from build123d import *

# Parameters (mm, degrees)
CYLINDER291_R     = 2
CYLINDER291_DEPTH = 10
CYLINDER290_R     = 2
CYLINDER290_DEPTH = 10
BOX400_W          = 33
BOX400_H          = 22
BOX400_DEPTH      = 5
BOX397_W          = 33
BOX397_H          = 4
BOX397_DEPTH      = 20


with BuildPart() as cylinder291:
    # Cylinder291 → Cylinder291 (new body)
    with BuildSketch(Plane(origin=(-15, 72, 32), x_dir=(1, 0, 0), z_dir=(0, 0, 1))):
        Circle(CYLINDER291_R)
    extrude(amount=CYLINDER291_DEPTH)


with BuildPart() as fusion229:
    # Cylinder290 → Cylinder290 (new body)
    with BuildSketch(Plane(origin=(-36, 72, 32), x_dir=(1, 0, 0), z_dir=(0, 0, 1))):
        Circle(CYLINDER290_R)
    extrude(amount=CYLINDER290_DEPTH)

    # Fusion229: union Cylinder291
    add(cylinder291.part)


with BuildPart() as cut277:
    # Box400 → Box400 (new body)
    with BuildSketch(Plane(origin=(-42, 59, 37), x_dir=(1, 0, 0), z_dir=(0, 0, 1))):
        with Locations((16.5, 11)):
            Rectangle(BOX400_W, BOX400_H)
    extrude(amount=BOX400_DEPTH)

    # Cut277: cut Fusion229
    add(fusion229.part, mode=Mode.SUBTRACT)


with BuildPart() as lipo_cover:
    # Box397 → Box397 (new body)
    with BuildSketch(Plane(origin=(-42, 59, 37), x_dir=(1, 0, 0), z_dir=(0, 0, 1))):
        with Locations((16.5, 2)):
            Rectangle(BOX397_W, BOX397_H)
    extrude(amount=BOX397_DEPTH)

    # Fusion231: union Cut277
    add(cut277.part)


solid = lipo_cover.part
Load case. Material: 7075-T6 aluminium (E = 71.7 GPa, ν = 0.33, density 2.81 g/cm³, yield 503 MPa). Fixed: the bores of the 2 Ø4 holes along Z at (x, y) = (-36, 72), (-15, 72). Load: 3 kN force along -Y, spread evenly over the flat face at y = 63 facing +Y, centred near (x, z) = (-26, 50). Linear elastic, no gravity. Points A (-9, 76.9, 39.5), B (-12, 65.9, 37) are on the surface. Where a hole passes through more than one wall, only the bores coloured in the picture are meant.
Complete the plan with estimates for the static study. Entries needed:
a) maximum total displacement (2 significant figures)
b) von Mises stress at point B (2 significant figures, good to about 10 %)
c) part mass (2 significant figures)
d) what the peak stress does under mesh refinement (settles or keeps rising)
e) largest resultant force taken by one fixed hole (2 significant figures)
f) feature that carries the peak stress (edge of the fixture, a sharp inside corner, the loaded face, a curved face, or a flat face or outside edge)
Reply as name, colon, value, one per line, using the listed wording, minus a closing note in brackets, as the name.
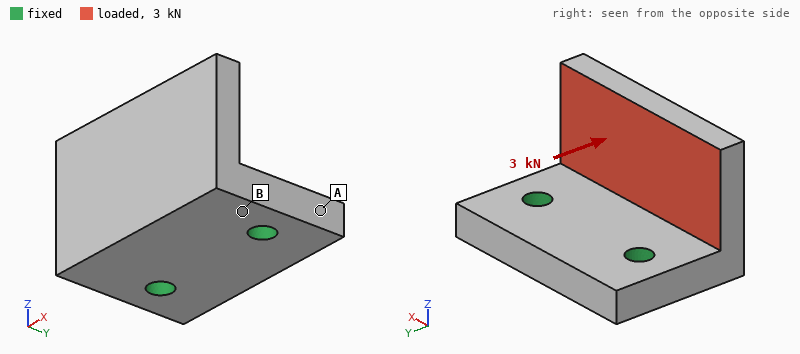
maximum total displacement: 0.37 mm
von Mises stress at point B: 200 MPa
part mass: 15 g
what the peak stress does under mesh refinement: keeps rising
largest resultant force taken by one fixed hole: 1.5 kN
feature that carries the peak stress: edge of the fixture
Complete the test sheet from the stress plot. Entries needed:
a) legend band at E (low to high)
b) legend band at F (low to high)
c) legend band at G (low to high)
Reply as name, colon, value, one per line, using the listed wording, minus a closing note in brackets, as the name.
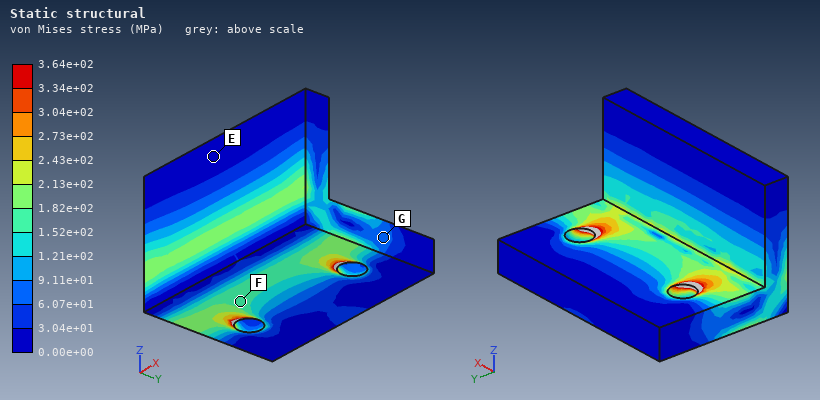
legend band at E: 0.00e+00 to 3.04e+01 MPa
legend band at F: 1.52e+02 to 1.82e+02 MPa
legend band at G: 6.07e+01 to 9.11e+01 MPa
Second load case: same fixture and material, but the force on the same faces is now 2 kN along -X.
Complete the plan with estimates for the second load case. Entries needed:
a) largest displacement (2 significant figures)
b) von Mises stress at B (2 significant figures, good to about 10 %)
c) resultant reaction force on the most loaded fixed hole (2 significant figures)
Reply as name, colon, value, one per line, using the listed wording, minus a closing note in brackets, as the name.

largest displacement: 78 µm
von Mises stress at B: 51 MPa
resultant reaction force on the most loaded fixed hole: 1.5 kN
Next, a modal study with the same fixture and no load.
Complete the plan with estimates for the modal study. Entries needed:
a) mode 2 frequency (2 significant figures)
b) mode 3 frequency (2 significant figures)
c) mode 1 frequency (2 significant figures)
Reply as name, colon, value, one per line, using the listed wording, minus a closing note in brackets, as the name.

mode 2 frequency: 12 kHz
mode 3 frequency: 17 kHz
mode 1 frequency: 6900 Hz
